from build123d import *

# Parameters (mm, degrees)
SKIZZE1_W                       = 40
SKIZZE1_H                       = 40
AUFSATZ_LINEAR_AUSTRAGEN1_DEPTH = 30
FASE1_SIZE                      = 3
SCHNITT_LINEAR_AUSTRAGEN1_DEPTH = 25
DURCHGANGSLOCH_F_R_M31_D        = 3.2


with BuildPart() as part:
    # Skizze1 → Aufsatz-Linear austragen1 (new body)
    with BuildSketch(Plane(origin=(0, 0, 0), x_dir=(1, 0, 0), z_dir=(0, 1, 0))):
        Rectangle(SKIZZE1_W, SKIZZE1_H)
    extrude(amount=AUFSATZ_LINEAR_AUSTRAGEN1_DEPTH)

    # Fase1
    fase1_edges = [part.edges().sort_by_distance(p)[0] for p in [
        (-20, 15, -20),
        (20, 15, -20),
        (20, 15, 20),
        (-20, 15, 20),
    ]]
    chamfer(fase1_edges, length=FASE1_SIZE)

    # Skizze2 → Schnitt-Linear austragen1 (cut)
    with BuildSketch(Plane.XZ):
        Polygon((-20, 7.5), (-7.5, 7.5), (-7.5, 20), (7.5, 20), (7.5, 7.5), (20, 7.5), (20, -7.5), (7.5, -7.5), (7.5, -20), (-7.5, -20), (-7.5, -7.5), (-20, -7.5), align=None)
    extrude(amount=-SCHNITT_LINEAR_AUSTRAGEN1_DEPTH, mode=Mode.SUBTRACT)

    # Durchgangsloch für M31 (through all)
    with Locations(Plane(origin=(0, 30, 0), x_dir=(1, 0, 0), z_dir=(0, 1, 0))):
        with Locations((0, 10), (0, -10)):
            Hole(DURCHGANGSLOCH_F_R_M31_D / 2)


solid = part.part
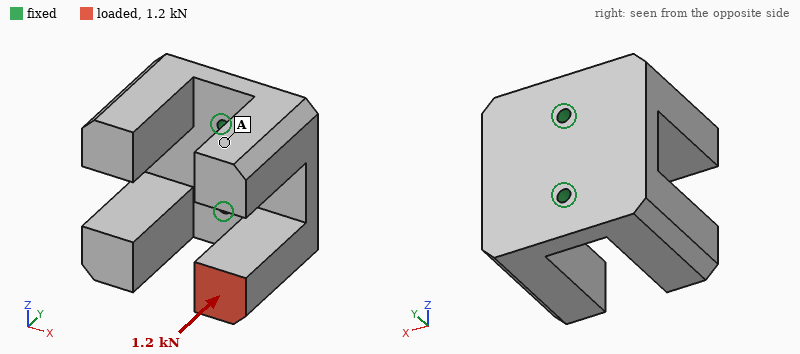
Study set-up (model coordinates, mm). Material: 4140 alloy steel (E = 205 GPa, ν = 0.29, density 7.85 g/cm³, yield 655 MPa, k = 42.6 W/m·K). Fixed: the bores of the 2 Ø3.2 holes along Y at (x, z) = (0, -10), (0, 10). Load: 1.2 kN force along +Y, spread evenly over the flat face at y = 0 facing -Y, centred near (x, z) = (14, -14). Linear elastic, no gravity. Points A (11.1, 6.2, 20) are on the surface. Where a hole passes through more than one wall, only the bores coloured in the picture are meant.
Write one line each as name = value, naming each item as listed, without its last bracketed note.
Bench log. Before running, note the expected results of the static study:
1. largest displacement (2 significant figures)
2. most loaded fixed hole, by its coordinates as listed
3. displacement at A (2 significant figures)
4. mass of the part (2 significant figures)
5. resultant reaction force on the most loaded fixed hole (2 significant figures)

largest displacement = 75 µm
most loaded fixed hole, by its coordinates as listed = (0, -10)
displacement at A = 20 µm
mass of the part = 180 g
resultant reaction force on the most loaded fixed hole = 1.2 kN
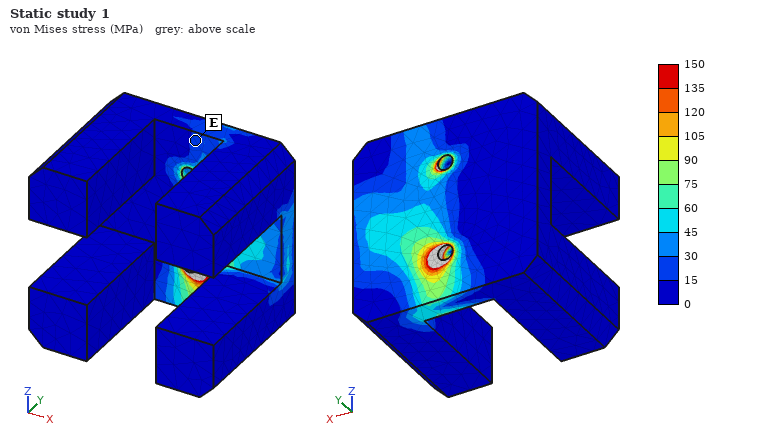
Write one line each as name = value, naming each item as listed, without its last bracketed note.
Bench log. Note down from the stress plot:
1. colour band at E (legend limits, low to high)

colour band at E = 15 to 30 MPa
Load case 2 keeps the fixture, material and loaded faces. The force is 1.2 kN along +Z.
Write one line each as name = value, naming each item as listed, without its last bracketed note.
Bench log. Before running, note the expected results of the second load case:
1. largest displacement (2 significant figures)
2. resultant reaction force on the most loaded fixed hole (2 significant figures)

largest displacement = 0.15 mm
resultant reaction force on the most loaded fixed hole = 1.4 kN
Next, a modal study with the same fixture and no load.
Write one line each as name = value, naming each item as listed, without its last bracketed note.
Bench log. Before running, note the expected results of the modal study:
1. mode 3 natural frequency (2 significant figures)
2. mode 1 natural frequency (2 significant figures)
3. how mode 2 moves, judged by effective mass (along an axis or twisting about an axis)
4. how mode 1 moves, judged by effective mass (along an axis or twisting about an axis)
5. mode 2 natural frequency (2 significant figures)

mode 3 natural frequency = 3400 Hz
mode 1 natural frequency = 2500 Hz
how mode 2 moves, judged by effective mass = along Y
how mode 1 moves, judged by effective mass = along X
mode 2 natural frequency = 3000 Hz
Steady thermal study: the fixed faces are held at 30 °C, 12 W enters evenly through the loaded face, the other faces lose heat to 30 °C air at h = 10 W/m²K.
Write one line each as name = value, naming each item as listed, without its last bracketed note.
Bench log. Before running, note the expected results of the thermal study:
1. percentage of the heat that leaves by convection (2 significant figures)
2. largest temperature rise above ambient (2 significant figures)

percentage of the heat that leaves by convection = 8.9 %
largest temperature rise above ambient = 75 K
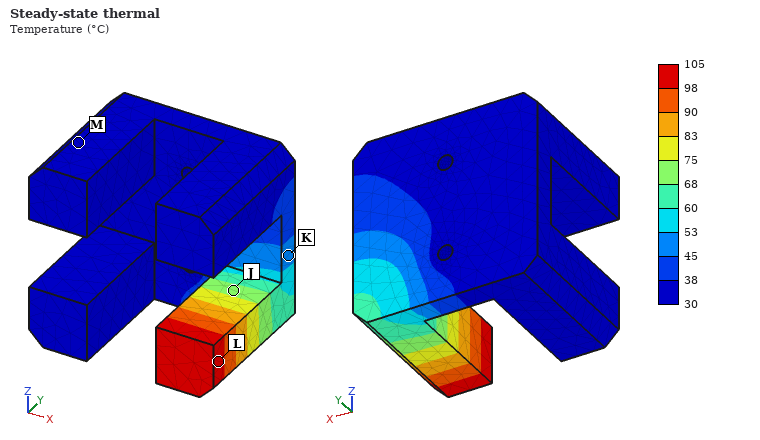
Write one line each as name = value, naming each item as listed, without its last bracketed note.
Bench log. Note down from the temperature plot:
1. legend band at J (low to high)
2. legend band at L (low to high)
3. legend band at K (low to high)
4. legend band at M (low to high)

legend band at J = 68 to 75 °C
legend band at L = 98 to 105 °C
legend band at K = 45 to 53 °C
legend band at M = 30 to 38 °C
